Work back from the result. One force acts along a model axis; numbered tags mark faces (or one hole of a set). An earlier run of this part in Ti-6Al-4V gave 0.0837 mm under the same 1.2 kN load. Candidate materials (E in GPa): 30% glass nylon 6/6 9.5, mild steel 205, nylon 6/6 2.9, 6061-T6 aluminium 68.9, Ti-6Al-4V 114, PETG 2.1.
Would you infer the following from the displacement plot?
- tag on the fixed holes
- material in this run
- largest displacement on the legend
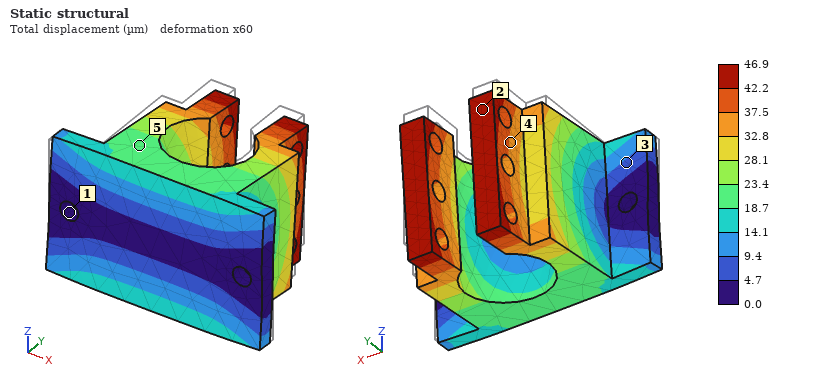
1
mild steel
46.9 µm
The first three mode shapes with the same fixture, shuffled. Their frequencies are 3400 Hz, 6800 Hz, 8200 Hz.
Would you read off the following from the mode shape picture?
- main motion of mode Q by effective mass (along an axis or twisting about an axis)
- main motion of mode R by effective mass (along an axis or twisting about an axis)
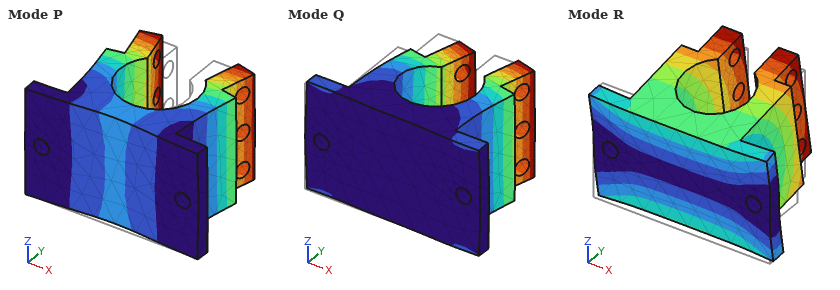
along X
along Z
